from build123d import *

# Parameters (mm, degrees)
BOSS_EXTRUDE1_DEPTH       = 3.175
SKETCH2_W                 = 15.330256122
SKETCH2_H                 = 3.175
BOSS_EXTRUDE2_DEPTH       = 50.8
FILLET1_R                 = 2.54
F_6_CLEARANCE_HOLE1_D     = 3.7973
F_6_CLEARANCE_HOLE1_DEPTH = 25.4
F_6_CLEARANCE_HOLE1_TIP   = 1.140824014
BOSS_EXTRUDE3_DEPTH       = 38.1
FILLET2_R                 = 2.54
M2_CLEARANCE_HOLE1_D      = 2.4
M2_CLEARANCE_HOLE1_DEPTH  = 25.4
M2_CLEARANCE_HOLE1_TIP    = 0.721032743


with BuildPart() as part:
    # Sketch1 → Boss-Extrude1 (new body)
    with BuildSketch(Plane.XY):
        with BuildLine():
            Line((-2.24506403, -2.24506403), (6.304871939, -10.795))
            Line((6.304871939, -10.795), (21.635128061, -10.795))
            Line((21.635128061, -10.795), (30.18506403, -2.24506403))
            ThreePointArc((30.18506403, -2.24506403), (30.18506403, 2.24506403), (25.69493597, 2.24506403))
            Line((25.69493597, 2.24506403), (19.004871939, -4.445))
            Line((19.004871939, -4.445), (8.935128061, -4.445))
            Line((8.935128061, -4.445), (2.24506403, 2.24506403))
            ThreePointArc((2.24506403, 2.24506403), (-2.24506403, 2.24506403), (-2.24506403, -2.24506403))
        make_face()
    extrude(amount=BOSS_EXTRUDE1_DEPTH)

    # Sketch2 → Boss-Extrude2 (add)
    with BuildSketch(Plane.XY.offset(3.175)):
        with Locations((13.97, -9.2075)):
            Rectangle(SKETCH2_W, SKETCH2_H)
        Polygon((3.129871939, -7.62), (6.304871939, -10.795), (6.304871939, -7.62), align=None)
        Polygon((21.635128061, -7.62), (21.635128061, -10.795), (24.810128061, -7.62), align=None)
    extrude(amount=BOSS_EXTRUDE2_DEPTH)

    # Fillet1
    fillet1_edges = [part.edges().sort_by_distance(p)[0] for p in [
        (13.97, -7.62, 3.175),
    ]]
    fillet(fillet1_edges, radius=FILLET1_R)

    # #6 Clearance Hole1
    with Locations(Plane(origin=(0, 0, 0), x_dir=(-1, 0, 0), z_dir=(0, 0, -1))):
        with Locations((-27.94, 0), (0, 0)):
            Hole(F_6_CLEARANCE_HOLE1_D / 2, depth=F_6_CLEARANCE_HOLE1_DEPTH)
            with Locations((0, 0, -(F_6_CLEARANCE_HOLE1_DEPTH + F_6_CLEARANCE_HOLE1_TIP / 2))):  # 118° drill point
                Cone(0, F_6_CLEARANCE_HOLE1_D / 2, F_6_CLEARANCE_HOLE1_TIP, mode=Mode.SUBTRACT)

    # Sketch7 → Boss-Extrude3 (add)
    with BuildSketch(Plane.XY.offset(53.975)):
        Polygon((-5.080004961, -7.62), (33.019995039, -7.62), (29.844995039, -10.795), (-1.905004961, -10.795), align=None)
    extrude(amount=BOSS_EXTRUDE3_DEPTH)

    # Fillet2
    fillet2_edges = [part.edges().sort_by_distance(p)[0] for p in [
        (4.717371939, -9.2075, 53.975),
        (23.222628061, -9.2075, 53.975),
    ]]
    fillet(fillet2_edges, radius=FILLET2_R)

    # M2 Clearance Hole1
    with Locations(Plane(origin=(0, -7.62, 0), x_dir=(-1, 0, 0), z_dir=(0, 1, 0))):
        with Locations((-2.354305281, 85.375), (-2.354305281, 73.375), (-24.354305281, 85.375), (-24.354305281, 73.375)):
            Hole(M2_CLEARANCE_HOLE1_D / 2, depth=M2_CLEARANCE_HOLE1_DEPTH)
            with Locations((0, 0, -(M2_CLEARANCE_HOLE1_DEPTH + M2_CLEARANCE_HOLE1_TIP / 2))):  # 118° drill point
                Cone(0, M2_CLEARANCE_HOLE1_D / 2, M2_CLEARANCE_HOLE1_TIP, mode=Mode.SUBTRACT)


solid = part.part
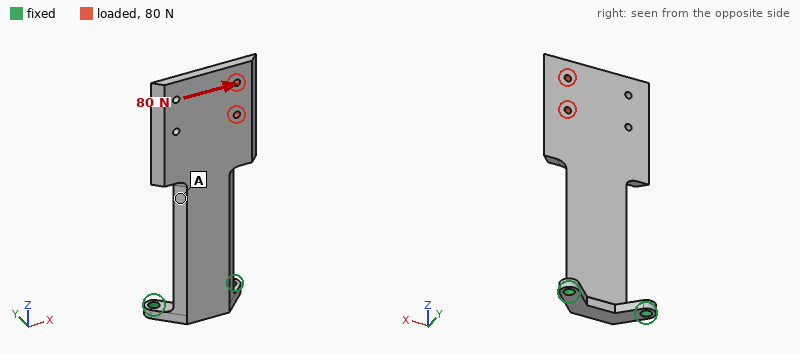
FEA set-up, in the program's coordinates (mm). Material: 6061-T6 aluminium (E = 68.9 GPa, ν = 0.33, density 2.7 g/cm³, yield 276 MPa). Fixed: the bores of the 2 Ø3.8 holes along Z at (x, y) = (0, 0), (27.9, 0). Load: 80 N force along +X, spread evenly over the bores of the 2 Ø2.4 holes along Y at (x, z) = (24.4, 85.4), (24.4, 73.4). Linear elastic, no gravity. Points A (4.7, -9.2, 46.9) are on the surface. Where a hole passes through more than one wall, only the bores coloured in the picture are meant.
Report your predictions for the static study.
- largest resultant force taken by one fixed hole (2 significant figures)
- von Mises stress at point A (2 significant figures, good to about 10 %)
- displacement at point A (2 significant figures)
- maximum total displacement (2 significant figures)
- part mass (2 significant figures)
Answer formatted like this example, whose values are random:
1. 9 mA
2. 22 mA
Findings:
1. 270 N
2. 14 MPa
3. 0.15 mm
4. 0.35 mm
5. 21 g
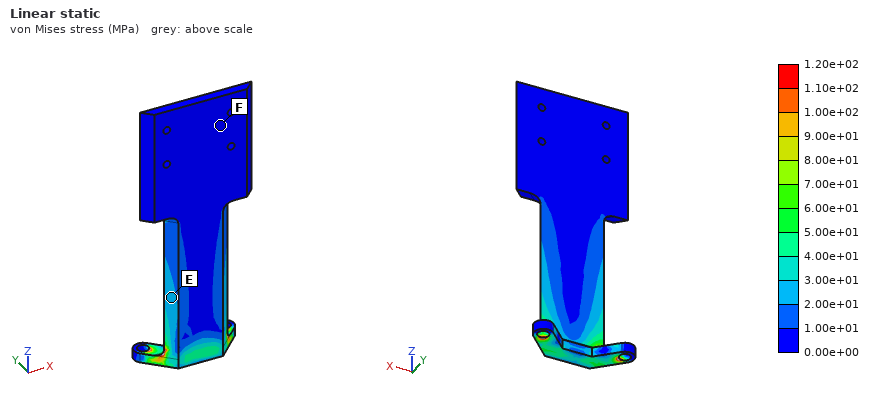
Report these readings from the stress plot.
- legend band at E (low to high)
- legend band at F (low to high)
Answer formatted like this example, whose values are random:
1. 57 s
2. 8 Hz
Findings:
1. 2.00e+01 to 3.00e+01 MPa
2. 0.00e+00 to 1.00e+01 MPa
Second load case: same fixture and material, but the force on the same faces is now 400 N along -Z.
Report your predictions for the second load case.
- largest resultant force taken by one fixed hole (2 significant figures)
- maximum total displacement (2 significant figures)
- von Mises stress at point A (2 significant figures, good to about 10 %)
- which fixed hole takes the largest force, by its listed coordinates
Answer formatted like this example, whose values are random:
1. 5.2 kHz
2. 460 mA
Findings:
1. 380 N
2. 0.79 mm
3. 15 MPa
4. (27.9, 0)
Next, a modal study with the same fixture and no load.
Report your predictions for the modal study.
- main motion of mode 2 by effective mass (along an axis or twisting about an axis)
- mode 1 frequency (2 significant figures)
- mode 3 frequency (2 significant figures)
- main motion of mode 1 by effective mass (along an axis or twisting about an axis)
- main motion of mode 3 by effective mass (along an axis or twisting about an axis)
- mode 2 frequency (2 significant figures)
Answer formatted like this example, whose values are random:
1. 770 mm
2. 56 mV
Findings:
1. along X
2. 200 Hz
3. 1300 Hz
4. along Y
5. twisting about Z
6. 820 Hz
